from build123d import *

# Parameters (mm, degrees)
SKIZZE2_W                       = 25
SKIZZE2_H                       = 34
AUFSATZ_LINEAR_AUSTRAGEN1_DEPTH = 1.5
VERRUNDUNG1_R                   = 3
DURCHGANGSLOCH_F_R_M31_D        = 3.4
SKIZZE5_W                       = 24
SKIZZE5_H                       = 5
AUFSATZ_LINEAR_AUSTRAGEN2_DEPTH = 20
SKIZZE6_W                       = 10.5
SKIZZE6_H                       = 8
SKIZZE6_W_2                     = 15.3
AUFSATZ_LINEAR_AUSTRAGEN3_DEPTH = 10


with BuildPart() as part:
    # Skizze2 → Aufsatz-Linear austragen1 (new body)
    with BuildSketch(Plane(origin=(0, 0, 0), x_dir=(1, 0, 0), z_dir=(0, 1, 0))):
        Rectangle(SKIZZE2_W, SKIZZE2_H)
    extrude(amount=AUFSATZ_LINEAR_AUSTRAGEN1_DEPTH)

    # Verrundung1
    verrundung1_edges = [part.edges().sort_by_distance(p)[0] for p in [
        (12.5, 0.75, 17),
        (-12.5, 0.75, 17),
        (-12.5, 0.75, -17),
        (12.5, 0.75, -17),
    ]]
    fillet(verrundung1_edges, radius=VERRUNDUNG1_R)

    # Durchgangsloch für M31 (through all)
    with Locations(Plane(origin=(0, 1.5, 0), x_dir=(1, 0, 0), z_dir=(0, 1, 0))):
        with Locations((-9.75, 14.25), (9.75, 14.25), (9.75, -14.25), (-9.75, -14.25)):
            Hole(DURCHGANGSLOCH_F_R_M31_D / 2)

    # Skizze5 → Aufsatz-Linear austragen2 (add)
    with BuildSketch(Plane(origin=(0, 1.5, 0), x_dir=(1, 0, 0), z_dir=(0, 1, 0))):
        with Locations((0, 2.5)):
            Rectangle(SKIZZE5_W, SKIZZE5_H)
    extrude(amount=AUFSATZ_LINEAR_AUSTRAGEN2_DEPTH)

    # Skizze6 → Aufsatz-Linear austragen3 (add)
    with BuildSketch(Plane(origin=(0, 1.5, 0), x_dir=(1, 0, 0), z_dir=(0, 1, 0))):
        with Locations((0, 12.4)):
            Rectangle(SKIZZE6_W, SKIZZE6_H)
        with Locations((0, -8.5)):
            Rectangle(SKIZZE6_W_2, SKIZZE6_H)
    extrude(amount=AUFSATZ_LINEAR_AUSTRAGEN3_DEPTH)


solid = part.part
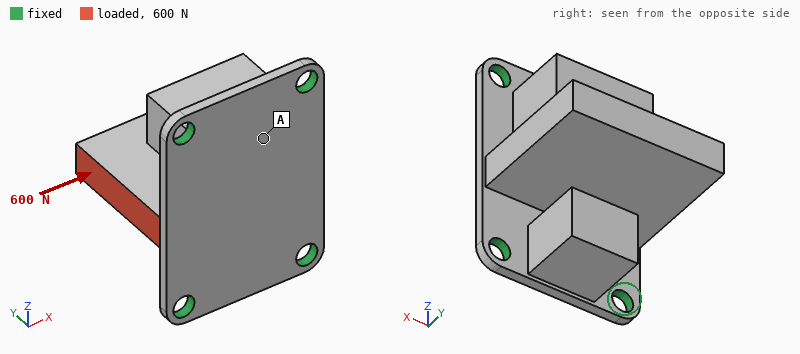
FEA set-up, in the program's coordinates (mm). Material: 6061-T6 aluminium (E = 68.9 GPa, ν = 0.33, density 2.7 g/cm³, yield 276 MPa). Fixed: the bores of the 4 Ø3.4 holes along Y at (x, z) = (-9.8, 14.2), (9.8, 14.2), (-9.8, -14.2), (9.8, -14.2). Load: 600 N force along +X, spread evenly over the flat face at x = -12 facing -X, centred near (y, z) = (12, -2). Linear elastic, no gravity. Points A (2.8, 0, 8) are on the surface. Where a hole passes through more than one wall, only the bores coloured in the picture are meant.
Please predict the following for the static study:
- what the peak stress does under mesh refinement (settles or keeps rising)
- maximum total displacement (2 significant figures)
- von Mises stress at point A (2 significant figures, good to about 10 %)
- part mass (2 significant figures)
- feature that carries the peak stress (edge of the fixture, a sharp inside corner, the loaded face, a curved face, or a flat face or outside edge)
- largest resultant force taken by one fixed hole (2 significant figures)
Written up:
keeps rising
0.12 mm
14 MPa
15 g
edge of the fixture
290 N
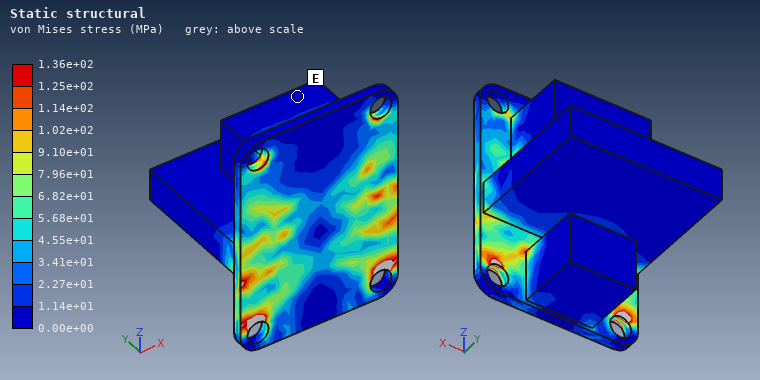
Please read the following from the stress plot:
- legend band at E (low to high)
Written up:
0.00e+00 to 1.14e+01 MPa
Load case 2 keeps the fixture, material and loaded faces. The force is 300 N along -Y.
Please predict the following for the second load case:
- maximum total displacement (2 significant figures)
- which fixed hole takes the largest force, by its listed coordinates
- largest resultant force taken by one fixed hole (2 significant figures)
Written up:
0.10 mm
(-9.8, -14.2)
210 N
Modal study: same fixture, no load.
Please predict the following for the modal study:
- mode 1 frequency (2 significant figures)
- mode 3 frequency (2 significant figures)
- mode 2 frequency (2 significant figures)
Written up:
3100 Hz
5000 Hz
4900 Hz
